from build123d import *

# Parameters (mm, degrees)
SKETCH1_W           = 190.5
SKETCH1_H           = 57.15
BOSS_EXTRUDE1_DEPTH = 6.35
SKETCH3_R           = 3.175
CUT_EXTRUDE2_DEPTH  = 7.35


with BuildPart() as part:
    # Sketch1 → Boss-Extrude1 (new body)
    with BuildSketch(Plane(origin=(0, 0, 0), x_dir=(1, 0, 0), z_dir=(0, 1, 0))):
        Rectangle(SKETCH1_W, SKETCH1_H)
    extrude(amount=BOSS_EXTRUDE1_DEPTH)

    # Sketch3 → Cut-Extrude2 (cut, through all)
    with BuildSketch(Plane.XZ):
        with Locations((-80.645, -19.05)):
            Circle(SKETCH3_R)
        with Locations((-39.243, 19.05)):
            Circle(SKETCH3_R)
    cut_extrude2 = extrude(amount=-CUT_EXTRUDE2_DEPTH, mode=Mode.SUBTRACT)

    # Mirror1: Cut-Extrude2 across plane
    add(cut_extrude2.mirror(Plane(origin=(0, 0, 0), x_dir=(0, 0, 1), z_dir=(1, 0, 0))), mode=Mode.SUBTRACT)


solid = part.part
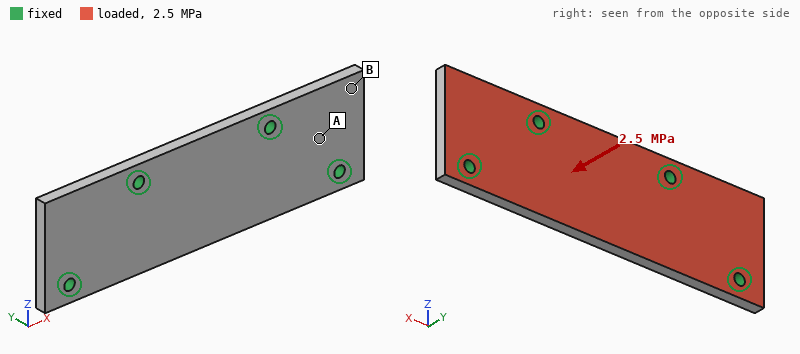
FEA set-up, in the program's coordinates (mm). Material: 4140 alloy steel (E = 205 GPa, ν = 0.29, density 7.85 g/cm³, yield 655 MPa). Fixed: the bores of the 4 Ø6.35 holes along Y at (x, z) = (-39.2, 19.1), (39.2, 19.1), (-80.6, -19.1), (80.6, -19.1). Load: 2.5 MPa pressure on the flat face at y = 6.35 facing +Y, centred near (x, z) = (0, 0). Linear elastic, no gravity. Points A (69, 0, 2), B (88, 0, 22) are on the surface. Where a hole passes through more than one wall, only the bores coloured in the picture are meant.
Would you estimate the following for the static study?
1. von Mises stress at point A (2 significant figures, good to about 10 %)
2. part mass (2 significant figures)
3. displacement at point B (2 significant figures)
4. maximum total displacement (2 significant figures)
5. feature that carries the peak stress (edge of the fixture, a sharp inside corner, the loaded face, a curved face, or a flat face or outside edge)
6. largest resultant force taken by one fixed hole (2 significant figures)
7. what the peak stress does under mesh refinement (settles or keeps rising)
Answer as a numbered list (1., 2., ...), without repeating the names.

1. 130 MPa
2. 540 g
3. 0.075 mm
4. 0.37 mm
5. edge of the fixture
6. 8.2 kN
7. keeps rising
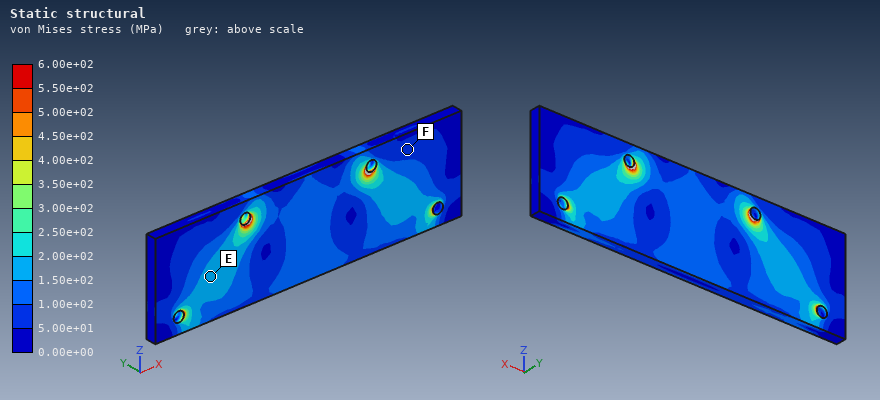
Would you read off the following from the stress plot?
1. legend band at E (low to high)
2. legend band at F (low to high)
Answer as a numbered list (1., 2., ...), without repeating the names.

1. 1.50e+02 to 2.00e+02 MPa
2. 5.00e+01 to 1.00e+02 MPa
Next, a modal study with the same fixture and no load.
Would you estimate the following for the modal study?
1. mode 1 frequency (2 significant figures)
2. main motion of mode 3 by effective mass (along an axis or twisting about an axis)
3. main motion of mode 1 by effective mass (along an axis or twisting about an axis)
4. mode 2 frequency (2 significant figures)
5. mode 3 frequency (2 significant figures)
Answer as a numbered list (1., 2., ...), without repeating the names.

1. 2400 Hz
2. along Y
3. along Y
4. 3800 Hz
5. 3900 Hz
